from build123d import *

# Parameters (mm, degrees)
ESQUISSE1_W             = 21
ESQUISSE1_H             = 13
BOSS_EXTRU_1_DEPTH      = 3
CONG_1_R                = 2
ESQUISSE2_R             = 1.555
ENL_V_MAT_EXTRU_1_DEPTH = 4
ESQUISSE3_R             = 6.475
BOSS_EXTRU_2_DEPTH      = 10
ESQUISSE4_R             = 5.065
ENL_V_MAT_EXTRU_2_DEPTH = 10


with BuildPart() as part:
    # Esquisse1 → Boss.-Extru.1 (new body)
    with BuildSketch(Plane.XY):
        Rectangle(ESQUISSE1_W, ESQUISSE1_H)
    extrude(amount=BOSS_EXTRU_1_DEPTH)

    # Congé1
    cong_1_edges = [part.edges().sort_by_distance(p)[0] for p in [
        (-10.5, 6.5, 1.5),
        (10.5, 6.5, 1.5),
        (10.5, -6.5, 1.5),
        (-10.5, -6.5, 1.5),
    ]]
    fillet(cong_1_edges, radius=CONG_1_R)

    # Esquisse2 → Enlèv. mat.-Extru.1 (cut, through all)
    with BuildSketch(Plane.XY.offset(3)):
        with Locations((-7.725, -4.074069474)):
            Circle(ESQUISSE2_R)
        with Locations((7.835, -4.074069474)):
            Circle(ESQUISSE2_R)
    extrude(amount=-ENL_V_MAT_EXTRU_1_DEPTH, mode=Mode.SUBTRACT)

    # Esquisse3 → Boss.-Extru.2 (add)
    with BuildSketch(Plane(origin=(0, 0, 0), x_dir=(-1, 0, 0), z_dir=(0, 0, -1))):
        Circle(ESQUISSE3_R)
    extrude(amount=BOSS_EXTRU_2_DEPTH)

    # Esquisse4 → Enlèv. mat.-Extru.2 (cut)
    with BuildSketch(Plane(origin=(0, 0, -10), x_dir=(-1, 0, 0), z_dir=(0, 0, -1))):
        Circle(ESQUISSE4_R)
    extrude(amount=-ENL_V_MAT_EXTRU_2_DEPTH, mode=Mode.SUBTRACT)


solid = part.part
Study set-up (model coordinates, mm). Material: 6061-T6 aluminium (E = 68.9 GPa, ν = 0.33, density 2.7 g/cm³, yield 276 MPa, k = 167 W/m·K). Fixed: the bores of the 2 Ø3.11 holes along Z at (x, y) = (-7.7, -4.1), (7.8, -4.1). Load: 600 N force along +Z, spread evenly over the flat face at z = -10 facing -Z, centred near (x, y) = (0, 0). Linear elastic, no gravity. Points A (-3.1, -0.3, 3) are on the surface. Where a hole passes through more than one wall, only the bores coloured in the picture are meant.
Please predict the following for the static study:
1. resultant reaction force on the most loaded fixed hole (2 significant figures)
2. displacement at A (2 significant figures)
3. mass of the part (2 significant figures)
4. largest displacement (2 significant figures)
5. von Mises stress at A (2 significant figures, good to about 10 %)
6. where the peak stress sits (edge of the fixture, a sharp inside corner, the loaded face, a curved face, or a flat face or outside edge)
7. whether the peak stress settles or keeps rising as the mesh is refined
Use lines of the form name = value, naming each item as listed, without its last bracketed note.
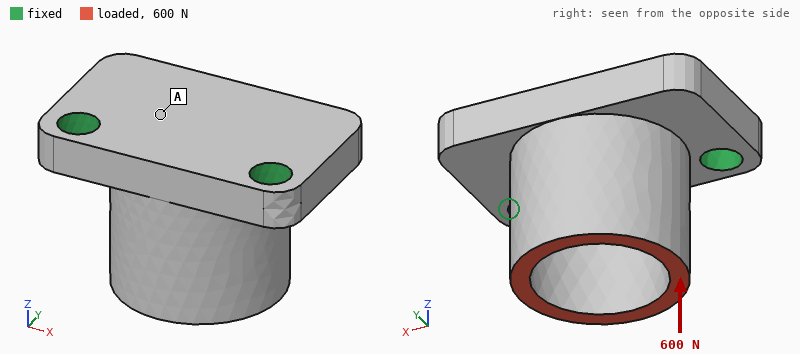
resultant reaction force on the most loaded fixed hole = 300 N
displacement at A = 7.3 µm
mass of the part = 3.4 g
largest displacement = 33 µm
von Mises stress at A = 17 MPa
where the peak stress sits = edge of the fixture
whether the peak stress settles or keeps rising as the mesh is refined = keeps rising
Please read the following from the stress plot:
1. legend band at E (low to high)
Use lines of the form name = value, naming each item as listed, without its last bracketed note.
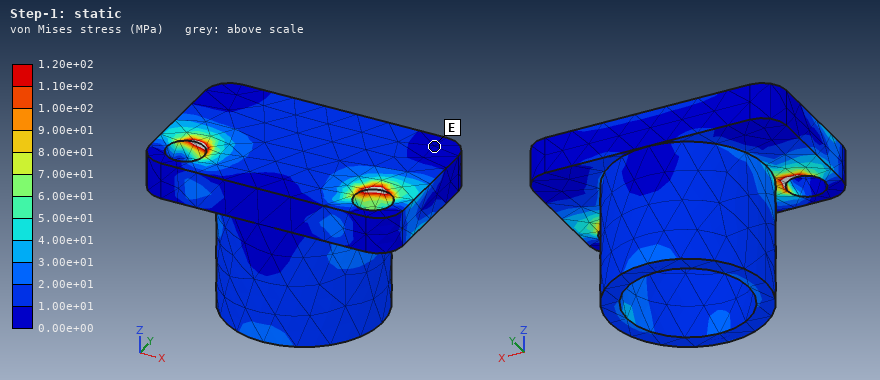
legend band at E = 0.00e+00 to 1.00e+01 MPa
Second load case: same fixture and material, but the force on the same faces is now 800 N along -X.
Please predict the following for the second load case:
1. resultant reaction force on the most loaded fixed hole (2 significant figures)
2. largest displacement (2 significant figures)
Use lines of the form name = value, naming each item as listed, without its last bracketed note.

resultant reaction force on the most loaded fixed hole = 810 N
largest displacement = 42 µm
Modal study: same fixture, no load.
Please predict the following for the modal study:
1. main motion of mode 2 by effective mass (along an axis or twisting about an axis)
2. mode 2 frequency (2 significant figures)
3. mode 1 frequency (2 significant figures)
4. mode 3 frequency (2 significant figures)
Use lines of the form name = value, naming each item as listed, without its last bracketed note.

main motion of mode 2 by effective mass = along X
mode 2 frequency = 28 kHz
mode 1 frequency = 13 kHz
mode 3 frequency = 34 kHz
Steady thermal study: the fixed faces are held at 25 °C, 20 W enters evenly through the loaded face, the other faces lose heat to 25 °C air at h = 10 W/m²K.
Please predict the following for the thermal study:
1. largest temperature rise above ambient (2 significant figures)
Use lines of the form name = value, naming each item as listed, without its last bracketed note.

largest temperature rise above ambient = 33 K
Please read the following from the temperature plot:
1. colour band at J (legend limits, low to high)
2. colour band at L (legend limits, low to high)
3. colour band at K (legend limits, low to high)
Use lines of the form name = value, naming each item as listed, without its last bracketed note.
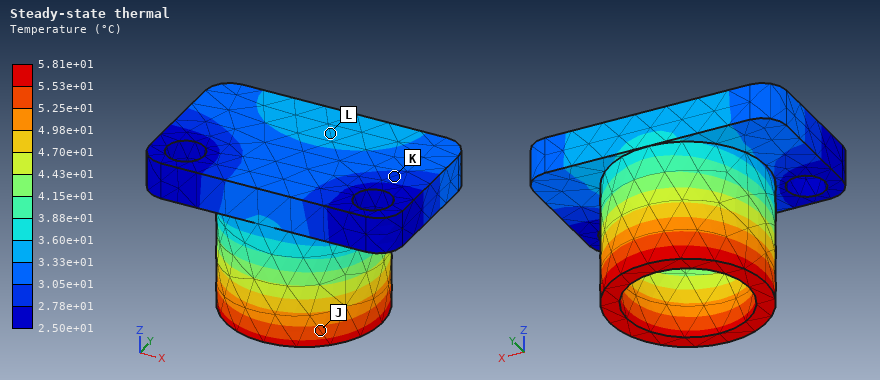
colour band at J = 5.25e+01 to 5.53e+01 °C
colour band at L = 3.33e+01 to 3.60e+01 °C
colour band at K = 2.78e+01 to 3.05e+01 °C
